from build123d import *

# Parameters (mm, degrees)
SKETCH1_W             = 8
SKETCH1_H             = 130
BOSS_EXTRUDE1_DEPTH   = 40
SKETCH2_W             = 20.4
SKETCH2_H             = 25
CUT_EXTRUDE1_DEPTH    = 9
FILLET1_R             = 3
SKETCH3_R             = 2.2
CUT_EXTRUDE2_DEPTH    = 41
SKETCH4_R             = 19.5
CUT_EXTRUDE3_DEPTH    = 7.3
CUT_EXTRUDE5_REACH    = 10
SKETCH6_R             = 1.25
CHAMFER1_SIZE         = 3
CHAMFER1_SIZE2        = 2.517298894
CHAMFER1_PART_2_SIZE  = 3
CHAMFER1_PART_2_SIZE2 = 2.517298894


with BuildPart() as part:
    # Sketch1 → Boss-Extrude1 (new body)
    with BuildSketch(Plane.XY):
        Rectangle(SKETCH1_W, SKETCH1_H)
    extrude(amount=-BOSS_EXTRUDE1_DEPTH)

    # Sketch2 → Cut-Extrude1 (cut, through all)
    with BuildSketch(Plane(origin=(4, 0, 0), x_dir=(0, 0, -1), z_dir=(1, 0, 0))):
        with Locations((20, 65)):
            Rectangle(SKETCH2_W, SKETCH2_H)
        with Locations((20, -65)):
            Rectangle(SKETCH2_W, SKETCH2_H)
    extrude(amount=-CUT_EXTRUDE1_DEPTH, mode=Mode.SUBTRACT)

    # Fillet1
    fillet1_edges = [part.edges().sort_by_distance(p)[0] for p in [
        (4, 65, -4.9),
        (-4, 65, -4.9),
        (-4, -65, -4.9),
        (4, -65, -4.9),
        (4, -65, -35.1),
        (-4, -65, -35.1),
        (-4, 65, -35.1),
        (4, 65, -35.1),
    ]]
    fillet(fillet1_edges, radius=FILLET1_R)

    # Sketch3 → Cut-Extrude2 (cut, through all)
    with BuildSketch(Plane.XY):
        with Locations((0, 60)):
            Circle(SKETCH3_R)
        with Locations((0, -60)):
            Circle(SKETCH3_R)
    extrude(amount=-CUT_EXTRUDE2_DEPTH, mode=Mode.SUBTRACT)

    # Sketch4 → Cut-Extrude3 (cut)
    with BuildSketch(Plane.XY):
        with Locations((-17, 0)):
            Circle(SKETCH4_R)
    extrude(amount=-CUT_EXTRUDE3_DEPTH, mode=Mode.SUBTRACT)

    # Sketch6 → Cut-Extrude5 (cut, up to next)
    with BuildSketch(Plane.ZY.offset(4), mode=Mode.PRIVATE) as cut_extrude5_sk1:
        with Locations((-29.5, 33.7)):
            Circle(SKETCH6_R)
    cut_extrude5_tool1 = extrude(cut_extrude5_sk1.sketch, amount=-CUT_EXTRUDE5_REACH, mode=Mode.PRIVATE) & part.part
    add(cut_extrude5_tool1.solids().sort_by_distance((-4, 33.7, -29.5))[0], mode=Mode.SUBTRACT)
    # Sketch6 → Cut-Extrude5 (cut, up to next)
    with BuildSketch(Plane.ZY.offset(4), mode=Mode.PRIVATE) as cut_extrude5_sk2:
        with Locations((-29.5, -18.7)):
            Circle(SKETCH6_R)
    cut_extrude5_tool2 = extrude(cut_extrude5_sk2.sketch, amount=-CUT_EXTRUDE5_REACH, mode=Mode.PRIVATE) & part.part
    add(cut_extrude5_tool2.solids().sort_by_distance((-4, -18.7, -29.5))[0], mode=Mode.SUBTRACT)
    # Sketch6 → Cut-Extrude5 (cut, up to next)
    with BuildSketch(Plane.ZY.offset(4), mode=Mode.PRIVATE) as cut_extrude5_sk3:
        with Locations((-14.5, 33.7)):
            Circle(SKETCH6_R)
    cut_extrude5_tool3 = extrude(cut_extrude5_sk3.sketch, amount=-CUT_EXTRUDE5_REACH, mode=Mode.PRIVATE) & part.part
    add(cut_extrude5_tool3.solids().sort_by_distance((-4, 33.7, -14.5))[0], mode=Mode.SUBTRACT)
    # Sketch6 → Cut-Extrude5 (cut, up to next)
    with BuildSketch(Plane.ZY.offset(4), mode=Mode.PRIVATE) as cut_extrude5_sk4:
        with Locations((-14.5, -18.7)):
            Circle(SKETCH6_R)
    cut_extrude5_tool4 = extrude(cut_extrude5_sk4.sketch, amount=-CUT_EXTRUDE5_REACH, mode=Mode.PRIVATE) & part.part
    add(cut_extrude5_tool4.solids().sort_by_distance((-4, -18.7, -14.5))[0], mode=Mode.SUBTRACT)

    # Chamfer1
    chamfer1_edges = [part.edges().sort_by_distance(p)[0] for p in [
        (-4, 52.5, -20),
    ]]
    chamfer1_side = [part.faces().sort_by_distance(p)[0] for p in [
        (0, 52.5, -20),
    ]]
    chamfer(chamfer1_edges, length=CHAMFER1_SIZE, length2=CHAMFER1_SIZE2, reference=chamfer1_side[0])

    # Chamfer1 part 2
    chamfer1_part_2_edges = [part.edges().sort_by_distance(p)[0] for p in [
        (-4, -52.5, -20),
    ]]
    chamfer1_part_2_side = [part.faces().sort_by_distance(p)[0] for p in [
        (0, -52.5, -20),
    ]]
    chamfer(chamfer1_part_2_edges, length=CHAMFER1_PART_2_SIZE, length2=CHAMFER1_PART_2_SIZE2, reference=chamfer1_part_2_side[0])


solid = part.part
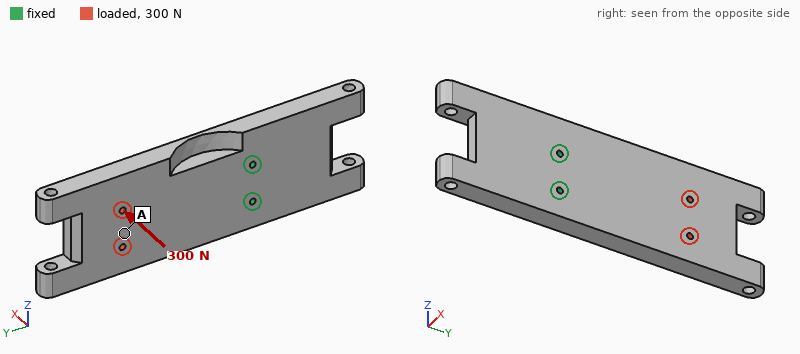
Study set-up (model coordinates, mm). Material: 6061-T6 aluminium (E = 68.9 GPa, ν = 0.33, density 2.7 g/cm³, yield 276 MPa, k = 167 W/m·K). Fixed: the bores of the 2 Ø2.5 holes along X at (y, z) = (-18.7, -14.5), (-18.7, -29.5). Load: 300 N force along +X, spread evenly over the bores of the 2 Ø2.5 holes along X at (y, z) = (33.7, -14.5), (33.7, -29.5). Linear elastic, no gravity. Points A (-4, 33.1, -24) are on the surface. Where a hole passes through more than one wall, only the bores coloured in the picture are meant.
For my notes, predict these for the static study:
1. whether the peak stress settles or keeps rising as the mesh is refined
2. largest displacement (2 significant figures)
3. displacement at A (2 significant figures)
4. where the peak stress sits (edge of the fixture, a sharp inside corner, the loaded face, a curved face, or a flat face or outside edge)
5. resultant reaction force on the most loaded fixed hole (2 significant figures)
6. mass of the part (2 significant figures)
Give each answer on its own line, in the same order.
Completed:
keeps rising
0.29 mm
0.16 mm
edge of the fixture
150 N
96 g
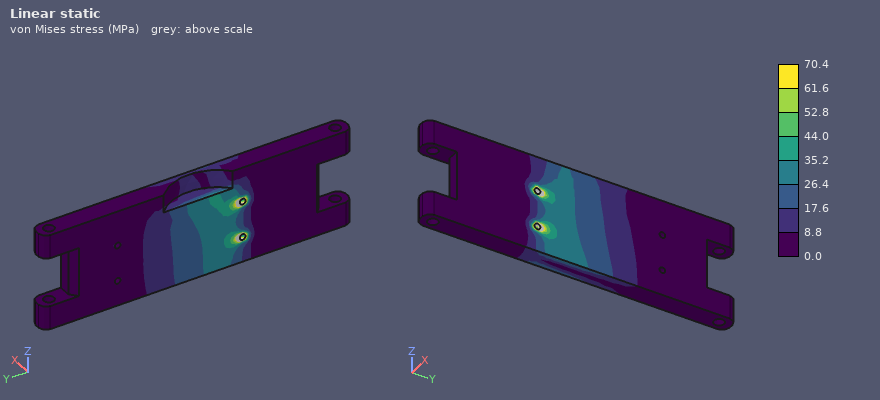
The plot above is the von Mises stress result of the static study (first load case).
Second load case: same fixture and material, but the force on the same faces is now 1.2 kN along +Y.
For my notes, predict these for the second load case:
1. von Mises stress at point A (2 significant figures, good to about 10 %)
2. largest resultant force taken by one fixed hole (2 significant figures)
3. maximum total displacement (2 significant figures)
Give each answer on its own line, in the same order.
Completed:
2.3 MPa
600 N
5.4 µm
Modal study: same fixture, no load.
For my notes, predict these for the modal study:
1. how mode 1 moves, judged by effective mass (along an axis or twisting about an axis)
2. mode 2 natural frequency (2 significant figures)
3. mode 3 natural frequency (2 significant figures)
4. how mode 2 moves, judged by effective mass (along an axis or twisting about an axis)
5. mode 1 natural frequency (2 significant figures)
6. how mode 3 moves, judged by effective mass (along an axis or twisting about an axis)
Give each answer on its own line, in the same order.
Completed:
along X
3100 Hz
3500 Hz
along Z
990 Hz
twisting about Y
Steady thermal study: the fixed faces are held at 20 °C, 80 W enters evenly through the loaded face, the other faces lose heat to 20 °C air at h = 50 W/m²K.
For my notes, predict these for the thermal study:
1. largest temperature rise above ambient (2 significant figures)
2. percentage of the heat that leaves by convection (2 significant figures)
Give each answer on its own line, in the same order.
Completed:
77 K
26 %
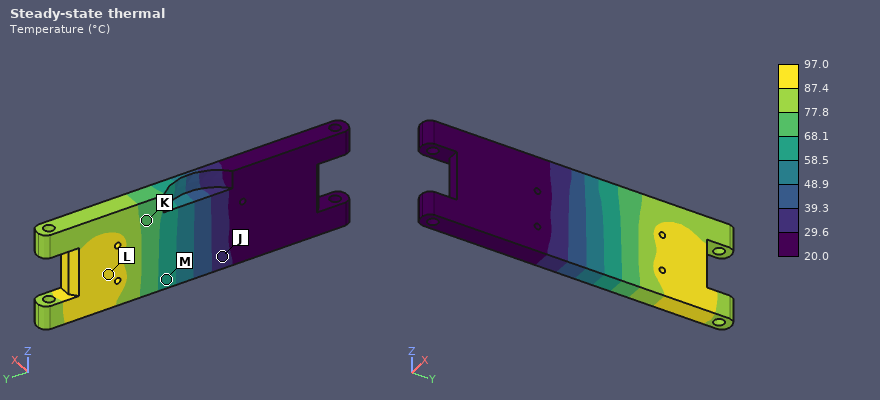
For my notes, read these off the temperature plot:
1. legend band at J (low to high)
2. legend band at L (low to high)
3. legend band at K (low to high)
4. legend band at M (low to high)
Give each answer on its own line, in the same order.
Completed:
29.6 to 39.3 °C
87.4 to 97.0 °C
68.1 to 77.8 °C
58.5 to 68.1 °C
